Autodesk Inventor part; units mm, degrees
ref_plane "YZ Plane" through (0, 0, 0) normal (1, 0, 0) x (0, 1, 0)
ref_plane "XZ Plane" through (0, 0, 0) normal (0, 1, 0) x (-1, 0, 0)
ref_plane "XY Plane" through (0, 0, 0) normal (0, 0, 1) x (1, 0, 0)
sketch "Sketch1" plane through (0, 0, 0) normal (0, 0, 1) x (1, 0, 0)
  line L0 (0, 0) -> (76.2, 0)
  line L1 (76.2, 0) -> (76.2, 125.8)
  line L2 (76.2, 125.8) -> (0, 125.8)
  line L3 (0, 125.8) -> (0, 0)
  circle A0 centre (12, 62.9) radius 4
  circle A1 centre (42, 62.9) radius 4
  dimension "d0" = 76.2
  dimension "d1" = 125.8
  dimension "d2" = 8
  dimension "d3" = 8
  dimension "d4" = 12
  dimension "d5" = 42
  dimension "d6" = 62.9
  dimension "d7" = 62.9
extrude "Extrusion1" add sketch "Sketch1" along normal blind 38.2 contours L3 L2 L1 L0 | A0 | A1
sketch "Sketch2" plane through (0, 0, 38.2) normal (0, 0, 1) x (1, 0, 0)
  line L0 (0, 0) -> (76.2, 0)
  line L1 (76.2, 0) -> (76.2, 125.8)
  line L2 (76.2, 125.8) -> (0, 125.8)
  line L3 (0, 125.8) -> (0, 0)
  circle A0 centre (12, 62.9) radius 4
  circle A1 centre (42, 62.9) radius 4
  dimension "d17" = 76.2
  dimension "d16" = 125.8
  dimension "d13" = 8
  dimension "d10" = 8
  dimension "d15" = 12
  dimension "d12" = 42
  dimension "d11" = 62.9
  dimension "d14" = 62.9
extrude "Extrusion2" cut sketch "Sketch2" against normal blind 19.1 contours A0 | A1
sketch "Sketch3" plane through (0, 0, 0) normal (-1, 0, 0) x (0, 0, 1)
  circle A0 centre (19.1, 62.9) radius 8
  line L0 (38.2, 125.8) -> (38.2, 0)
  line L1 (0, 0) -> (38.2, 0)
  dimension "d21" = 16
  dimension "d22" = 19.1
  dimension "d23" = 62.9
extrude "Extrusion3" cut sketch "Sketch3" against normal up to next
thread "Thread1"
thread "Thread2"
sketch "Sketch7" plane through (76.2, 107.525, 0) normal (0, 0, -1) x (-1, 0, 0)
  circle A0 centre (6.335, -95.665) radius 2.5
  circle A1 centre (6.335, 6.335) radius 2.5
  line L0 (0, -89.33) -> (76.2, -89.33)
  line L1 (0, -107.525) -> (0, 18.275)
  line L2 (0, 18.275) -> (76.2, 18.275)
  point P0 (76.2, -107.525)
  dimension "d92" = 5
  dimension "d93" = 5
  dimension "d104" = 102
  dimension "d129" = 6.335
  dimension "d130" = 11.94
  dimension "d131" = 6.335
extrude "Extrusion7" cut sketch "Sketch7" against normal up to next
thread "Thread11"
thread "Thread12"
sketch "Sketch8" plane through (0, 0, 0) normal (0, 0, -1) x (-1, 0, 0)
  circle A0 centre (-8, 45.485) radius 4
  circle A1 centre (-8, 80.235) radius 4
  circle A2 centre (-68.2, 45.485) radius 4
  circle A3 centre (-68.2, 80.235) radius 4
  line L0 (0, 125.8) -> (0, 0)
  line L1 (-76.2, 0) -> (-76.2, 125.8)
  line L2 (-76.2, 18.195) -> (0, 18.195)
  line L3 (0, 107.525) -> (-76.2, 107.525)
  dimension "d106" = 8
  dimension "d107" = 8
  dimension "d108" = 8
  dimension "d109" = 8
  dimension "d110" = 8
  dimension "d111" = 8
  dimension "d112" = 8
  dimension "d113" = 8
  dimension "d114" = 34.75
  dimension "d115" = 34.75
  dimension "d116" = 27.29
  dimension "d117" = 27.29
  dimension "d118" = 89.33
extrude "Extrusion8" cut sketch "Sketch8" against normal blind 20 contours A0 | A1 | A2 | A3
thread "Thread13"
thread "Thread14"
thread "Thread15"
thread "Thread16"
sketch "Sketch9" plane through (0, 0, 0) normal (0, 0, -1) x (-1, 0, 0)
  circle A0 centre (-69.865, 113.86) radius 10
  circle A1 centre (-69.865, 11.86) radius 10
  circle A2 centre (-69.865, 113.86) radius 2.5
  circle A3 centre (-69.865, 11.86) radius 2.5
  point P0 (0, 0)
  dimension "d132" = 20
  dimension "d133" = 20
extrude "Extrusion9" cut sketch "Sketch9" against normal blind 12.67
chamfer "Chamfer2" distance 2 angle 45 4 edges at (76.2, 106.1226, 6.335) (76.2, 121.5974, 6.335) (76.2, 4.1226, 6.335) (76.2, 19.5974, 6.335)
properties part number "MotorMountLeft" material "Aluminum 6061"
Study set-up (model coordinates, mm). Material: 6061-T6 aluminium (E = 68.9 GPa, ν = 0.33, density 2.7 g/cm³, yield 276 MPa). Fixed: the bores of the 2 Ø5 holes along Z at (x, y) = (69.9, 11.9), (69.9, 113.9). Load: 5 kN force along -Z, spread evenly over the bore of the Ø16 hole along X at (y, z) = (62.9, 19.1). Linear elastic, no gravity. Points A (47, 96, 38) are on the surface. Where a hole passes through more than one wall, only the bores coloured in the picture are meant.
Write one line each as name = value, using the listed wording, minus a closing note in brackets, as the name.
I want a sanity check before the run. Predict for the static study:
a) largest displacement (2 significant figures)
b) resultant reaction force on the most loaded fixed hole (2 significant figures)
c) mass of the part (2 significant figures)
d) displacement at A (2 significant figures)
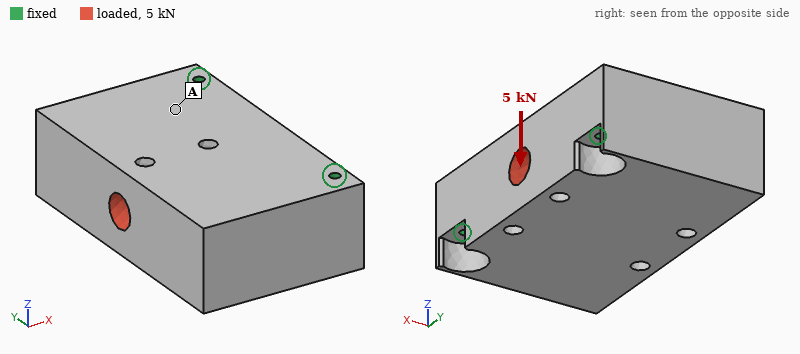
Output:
largest displacement = 49 µm
resultant reaction force on the most loaded fixed hole = 2.5 kN
mass of the part = 910 g
displacement at A = 16 µm
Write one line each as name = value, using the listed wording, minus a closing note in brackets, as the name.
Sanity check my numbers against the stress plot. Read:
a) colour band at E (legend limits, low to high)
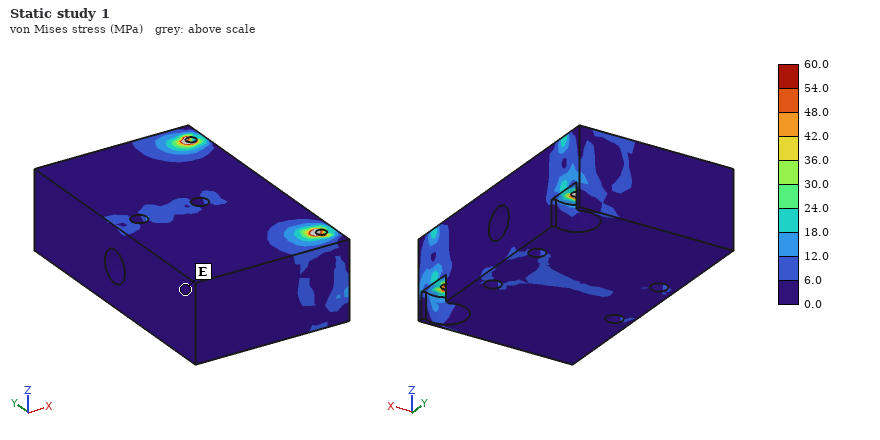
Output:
colour band at E = 0.0 to 6.0 MPa
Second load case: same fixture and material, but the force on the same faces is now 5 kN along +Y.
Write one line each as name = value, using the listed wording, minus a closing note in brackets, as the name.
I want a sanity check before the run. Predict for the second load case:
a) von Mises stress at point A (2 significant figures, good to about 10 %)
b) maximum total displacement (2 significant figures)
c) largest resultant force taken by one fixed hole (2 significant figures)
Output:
von Mises stress at point A = 2.2 MPa
maximum total displacement = 4.3 µm
largest resultant force taken by one fixed hole = 2.9 kN
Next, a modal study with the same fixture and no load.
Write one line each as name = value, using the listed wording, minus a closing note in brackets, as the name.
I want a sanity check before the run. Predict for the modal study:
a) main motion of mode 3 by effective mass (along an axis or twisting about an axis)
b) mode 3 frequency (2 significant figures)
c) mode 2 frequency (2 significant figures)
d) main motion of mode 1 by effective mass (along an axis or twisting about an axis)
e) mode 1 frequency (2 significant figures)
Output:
main motion of mode 3 by effective mass = along Y
mode 3 frequency = 6600 Hz
mode 2 frequency = 5400 Hz
main motion of mode 1 by effective mass = along Z
mode 1 frequency = 2100 Hz
